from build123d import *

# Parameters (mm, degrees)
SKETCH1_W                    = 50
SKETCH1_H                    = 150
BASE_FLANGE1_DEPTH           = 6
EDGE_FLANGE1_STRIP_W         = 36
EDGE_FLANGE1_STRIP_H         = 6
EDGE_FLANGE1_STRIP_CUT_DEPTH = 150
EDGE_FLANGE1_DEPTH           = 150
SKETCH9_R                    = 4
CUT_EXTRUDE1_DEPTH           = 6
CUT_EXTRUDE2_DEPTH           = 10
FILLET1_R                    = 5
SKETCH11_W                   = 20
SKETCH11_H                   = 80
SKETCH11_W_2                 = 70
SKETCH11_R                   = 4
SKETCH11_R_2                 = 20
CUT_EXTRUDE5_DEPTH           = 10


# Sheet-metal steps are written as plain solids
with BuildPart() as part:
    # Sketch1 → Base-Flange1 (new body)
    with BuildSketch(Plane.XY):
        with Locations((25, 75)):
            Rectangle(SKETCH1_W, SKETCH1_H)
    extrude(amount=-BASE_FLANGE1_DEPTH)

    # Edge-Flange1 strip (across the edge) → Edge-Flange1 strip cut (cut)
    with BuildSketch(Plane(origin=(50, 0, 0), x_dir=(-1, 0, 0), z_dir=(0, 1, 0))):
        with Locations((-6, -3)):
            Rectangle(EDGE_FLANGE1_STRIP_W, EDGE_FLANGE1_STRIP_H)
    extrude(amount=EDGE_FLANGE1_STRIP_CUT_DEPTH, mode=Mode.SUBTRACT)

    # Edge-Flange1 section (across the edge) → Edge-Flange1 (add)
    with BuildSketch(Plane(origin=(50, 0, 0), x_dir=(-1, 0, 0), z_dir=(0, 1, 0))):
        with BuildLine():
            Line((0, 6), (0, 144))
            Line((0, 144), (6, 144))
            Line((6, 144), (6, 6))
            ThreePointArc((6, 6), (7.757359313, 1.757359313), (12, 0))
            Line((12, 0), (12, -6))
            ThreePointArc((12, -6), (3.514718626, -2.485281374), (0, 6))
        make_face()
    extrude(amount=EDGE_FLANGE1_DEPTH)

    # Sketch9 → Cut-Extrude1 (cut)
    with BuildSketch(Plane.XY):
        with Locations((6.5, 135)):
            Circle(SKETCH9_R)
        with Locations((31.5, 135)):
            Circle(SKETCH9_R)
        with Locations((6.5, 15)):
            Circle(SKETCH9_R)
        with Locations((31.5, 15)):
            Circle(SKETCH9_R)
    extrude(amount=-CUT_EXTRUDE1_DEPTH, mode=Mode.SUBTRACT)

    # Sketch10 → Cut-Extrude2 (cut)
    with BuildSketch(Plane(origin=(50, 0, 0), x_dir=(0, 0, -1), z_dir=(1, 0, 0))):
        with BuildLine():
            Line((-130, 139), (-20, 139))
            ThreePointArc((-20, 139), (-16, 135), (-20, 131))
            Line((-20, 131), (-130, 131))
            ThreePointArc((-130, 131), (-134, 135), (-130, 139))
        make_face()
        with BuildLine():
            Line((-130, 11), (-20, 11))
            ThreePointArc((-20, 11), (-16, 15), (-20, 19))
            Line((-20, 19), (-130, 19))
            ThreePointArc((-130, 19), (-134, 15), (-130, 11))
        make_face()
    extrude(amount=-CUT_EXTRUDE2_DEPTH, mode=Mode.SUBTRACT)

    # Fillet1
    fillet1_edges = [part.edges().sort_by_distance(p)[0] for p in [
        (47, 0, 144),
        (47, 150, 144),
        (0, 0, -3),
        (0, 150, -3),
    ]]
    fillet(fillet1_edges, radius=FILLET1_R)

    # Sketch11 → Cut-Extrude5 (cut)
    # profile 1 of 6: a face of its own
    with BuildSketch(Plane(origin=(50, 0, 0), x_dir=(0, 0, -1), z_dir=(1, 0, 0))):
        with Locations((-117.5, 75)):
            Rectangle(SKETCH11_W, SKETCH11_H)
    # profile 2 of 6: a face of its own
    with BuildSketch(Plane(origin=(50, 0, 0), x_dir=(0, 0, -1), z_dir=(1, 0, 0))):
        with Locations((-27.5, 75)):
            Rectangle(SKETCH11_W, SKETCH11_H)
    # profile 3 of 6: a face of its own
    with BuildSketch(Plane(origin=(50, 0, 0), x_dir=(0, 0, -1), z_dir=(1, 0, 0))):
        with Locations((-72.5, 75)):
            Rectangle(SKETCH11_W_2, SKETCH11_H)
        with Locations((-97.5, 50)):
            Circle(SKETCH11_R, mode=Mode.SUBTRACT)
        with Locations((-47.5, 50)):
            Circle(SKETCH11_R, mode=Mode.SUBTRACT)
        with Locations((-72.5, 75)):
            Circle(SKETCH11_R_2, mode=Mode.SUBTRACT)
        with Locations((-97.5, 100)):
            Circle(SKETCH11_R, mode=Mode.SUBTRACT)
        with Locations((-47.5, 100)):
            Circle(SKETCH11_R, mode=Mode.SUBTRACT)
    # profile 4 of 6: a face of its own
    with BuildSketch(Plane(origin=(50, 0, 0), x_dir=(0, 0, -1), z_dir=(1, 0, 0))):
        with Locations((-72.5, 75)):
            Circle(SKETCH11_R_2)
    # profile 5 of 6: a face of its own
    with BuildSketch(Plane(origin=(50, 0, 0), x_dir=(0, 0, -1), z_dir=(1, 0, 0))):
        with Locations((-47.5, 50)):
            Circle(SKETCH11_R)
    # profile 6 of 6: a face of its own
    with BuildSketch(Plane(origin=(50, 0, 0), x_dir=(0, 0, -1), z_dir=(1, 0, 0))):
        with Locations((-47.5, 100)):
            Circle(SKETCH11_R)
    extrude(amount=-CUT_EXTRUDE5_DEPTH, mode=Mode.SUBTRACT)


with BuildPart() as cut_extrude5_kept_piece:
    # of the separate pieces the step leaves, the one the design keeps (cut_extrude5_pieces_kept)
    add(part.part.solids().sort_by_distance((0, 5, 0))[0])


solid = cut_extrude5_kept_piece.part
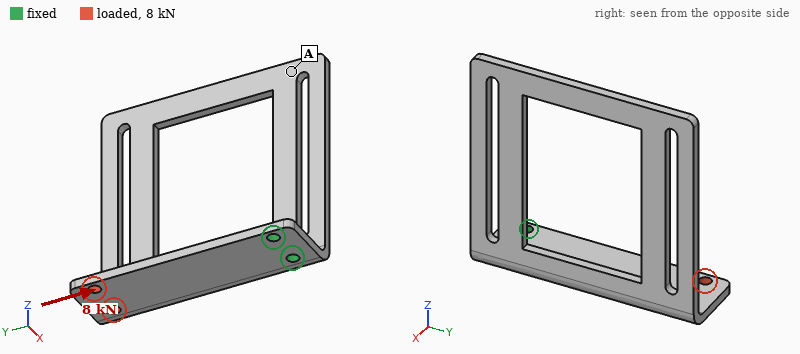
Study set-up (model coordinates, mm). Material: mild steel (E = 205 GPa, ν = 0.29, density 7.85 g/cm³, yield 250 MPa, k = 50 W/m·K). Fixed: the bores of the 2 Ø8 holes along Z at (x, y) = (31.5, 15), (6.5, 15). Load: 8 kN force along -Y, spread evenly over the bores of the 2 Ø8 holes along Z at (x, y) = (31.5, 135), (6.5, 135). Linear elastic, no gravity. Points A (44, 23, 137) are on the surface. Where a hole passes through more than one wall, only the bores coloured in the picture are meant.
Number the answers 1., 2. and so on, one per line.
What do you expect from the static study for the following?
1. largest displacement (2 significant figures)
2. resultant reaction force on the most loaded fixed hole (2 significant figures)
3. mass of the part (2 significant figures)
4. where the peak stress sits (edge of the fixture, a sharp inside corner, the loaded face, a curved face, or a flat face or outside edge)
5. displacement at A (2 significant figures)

1. 44 µm
2. 4.1 kN
3. 830 g
4. the loaded face
5. 9.2 µm
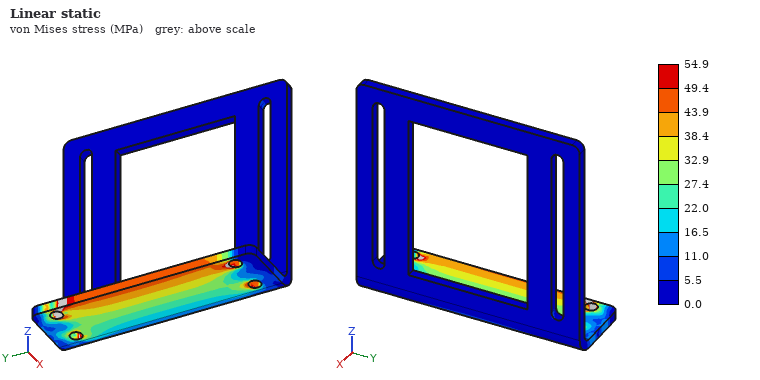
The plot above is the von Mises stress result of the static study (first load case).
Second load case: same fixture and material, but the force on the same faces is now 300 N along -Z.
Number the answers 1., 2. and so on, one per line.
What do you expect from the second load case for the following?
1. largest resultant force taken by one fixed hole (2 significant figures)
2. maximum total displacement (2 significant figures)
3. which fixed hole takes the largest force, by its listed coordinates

1. 240 N
2. 0.34 mm
3. (31.5, 15)
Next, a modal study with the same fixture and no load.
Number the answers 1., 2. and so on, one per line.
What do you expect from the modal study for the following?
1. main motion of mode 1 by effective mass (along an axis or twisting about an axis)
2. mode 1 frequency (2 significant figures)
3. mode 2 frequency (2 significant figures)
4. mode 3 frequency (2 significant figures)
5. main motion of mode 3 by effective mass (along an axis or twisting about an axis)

1. along X
2. 150 Hz
3. 240 Hz
4. 370 Hz
5. twisting about Z
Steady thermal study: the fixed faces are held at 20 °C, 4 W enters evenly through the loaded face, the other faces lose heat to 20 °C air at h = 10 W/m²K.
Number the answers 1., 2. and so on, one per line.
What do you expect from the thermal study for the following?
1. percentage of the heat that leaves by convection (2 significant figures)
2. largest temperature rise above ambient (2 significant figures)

1. 56 %
2. 18 K
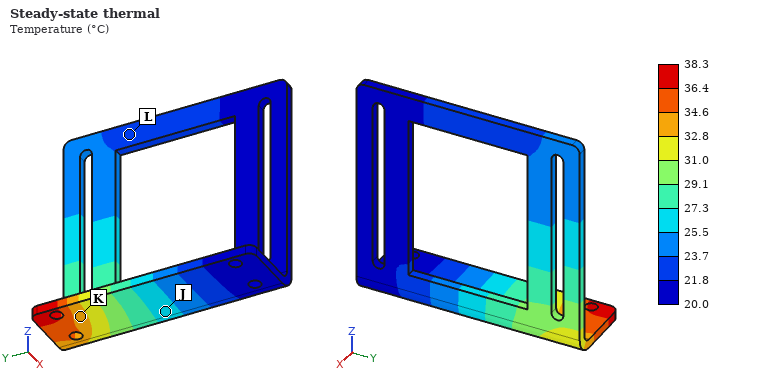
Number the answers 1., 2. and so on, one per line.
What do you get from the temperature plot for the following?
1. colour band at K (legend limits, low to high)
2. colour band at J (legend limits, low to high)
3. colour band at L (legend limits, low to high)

1. 32.8 to 34.6 °C
2. 25.5 to 27.3 °C
3. 21.8 to 23.7 °C
